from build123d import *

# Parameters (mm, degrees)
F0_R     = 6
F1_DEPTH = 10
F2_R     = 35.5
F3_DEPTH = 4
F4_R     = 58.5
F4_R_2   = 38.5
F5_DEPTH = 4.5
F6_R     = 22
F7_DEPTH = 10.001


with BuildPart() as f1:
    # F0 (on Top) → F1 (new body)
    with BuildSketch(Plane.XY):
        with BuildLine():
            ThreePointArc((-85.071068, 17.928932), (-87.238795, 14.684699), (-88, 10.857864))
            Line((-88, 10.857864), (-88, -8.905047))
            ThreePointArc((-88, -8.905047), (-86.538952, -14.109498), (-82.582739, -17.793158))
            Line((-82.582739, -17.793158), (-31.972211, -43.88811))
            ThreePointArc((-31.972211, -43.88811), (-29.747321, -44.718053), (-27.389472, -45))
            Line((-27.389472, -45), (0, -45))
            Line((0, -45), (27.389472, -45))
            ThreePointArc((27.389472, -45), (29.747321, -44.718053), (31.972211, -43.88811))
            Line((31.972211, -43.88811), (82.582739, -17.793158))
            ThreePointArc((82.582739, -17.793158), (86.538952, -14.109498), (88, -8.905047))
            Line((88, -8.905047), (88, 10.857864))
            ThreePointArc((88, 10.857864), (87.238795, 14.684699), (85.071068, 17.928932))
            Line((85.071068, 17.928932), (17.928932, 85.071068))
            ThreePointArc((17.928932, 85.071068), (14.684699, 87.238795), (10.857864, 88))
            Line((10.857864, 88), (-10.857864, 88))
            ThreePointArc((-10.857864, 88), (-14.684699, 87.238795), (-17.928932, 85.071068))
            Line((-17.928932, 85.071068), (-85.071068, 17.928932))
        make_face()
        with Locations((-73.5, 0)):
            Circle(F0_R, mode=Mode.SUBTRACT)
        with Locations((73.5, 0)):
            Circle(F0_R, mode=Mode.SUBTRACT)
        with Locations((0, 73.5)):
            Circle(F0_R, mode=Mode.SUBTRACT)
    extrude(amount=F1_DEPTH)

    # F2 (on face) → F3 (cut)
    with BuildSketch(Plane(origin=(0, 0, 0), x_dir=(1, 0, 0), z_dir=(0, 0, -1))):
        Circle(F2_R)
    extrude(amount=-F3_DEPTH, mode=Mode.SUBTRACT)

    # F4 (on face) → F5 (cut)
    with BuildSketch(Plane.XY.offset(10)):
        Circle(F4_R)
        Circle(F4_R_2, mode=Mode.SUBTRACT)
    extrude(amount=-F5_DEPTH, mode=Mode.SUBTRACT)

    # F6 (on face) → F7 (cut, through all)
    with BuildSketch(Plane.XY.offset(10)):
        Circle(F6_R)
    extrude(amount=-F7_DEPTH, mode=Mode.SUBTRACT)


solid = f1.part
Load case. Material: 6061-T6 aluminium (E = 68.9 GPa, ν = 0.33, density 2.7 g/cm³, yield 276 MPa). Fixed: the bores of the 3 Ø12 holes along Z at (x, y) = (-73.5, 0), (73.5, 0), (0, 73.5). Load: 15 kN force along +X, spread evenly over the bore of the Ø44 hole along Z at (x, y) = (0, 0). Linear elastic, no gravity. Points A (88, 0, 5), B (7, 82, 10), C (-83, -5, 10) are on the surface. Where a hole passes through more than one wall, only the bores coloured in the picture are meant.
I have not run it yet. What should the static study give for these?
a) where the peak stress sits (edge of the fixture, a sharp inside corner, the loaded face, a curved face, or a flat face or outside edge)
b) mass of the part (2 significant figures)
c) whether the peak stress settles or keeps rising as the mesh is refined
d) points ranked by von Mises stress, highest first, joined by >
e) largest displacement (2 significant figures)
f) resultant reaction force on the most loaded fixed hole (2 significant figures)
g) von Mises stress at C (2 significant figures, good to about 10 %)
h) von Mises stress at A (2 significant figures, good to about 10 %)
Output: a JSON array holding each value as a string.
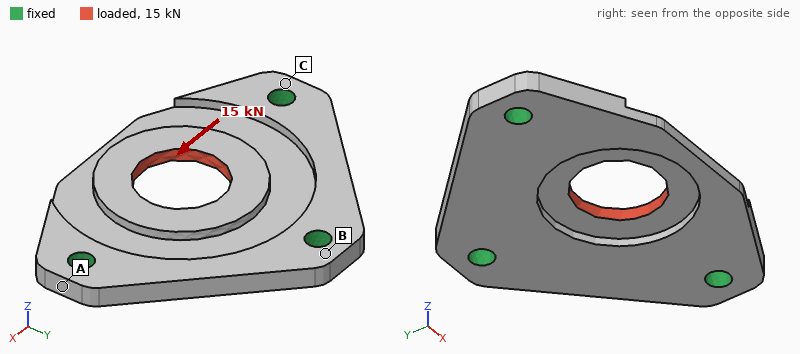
["edge of the fixture", "300 g", "keeps rising", "A > C > B", "36 µm", "6.2 kN", "10 MPa", "16 MPa"]
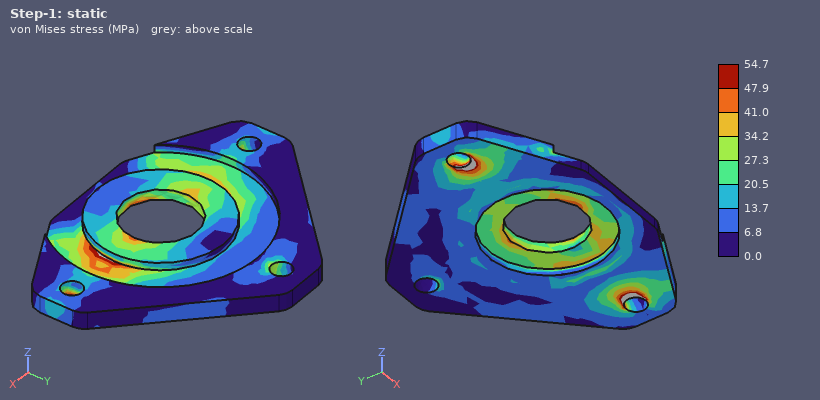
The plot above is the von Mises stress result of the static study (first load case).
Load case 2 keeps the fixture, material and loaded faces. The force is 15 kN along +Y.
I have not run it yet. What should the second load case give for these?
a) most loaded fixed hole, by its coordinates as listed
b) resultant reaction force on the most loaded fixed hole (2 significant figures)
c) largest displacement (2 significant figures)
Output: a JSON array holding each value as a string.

["(0, 73.5)", "6.6 kN", "0.15 mm"]
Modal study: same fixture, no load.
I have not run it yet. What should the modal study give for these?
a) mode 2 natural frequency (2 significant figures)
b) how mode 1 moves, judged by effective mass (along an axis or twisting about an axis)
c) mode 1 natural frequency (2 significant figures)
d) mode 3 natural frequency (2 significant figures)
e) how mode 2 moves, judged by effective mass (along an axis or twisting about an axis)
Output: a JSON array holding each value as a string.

["4200 Hz", "along Z", "2000 Hz", "4500 Hz", "along Z"]
